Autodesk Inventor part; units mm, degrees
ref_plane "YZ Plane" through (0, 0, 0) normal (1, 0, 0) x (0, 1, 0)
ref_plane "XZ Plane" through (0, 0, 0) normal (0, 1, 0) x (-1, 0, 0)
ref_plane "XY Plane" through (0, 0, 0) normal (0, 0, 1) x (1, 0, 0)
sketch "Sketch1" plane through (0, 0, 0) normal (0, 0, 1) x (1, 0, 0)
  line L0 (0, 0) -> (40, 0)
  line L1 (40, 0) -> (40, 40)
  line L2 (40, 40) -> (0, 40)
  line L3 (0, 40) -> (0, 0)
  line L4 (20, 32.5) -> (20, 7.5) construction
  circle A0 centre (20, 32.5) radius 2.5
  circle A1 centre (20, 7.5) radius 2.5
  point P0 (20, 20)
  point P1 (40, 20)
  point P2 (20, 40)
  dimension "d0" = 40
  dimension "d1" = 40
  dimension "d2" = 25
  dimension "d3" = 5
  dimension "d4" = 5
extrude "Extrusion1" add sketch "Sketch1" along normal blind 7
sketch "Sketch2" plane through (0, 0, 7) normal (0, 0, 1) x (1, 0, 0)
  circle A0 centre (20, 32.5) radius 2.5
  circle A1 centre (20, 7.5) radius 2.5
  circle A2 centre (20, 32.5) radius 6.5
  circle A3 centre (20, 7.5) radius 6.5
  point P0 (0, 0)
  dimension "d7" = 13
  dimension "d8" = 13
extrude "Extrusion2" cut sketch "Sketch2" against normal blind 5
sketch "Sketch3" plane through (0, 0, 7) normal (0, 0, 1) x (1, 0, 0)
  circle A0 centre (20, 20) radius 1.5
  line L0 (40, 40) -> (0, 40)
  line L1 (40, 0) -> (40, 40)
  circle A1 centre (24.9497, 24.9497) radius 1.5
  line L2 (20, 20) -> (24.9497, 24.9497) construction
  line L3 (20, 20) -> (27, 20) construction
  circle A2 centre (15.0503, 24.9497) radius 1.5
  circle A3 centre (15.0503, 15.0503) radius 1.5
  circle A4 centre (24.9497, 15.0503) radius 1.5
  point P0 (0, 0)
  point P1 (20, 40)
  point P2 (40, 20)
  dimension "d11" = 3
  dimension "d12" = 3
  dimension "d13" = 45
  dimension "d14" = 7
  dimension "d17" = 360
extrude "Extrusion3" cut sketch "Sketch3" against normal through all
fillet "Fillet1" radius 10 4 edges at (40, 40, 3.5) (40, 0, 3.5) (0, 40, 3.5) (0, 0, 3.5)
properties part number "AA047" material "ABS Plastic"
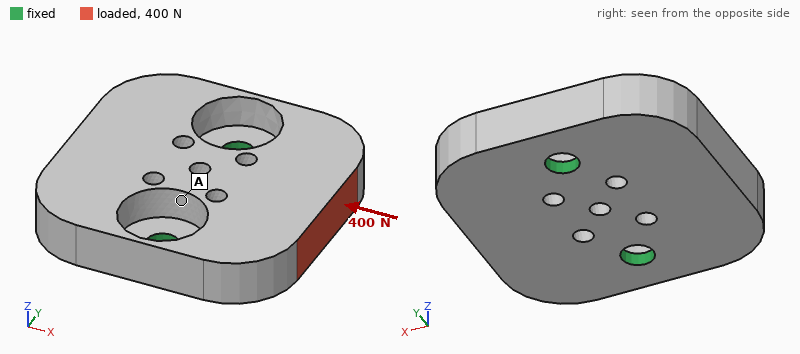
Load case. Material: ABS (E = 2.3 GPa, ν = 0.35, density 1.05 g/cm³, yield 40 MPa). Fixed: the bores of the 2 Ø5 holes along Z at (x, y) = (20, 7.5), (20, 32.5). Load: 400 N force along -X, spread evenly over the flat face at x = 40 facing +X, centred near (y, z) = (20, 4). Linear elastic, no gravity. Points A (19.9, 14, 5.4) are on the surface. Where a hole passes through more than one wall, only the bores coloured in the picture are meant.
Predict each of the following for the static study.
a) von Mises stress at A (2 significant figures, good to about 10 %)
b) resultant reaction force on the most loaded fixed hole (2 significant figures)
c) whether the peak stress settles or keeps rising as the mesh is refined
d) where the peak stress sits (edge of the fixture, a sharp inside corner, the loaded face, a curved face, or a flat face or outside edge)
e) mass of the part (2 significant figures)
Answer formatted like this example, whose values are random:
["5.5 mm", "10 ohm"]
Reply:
["4.1 MPa", "200 N", "keeps rising", "edge of the fixture", "9.4 g"]
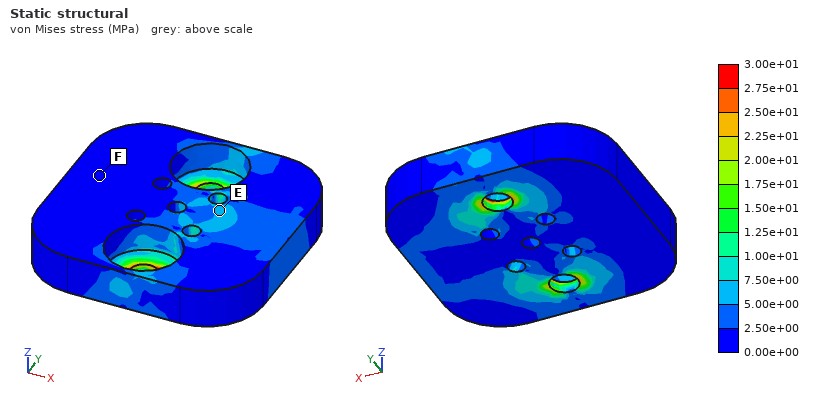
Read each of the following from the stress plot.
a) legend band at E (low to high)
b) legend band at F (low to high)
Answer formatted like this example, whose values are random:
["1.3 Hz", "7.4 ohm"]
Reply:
["5.00e+00 to 7.50e+00 MPa", "0.00e+00 to 2.50e+00 MPa"]
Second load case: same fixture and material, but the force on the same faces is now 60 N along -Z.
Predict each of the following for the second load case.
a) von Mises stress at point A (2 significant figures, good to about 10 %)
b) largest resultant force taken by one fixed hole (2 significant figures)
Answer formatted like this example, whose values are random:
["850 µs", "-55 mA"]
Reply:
["3.6 MPa", "37 N"]
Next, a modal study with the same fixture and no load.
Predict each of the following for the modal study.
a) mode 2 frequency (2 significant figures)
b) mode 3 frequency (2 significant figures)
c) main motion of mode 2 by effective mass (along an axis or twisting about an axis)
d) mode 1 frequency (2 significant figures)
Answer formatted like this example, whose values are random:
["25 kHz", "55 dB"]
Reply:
["2700 Hz", "3800 Hz", "along Z", "1100 Hz"]
